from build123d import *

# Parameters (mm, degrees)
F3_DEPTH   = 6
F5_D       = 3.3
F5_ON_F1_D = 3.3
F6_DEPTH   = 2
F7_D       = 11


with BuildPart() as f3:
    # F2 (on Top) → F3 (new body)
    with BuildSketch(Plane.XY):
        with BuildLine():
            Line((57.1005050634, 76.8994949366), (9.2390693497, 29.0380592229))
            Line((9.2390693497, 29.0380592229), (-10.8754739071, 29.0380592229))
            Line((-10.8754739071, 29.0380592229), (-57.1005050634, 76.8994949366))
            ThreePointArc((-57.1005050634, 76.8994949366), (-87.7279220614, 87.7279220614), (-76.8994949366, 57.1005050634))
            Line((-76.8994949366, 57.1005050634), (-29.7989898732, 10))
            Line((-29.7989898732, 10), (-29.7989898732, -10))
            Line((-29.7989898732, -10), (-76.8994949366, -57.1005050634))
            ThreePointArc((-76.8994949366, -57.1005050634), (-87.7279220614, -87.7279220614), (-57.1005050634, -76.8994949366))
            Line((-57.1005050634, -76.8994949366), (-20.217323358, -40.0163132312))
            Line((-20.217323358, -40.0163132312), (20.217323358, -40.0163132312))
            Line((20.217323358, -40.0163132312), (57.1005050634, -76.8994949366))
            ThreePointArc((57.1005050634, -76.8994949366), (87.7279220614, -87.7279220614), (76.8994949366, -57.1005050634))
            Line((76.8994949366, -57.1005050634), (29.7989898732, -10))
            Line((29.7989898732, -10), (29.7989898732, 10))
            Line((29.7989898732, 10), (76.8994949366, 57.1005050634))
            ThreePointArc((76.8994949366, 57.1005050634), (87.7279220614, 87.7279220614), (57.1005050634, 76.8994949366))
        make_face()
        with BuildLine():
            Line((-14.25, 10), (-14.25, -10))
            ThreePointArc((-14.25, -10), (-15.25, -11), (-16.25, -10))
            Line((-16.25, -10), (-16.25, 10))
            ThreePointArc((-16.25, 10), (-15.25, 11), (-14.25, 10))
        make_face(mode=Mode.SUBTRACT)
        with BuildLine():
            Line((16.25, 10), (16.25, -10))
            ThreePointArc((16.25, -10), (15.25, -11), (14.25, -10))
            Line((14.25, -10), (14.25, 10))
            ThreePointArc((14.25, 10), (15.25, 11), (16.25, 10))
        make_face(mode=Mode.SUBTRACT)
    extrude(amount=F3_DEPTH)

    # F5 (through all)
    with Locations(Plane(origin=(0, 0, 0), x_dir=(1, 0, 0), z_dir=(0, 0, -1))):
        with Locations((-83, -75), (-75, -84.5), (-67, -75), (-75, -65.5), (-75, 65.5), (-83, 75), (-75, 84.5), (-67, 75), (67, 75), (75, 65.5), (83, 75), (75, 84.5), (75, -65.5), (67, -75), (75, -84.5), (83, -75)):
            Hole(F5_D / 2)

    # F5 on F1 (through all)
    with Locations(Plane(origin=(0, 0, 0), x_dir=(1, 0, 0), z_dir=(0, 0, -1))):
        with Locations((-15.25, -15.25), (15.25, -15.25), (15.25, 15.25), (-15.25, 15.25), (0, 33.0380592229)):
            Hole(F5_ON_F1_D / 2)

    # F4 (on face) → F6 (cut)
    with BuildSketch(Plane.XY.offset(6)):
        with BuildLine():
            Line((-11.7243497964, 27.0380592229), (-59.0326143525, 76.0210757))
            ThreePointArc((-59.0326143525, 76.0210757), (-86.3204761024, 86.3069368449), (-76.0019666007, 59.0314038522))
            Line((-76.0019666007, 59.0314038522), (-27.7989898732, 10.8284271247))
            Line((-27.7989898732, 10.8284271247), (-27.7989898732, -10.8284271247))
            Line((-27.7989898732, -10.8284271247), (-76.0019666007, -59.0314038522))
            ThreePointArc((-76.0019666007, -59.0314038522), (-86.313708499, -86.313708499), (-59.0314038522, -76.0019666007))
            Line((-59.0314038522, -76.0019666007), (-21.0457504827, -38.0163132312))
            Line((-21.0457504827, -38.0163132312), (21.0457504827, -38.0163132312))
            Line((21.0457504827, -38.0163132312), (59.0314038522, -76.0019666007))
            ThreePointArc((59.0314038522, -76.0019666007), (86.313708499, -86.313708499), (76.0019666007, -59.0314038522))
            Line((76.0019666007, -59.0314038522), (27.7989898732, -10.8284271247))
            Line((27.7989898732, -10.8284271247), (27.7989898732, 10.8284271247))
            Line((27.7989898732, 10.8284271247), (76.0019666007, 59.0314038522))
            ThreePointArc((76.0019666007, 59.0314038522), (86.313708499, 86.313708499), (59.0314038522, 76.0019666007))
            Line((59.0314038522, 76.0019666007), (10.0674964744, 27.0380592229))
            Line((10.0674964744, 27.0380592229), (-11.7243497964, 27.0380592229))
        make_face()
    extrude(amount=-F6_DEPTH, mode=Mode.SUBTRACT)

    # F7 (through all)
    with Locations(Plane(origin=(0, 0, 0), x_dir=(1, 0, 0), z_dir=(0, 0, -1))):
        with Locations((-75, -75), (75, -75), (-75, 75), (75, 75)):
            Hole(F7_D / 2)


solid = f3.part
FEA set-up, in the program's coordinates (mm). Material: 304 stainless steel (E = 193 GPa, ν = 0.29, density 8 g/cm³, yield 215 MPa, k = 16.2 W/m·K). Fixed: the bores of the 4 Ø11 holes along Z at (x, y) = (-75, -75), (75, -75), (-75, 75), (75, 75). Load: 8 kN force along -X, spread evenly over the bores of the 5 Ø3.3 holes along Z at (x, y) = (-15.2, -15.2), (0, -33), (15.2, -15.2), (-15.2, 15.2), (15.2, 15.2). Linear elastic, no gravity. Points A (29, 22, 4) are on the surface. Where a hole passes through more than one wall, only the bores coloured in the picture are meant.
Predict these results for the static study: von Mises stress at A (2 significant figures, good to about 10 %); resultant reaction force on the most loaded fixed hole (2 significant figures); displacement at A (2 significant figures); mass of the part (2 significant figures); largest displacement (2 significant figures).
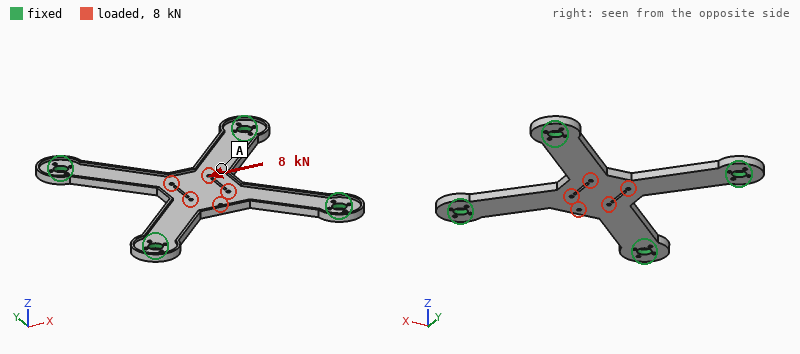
18 MPa
2.8 kN
11 µm
460 g
17 µm
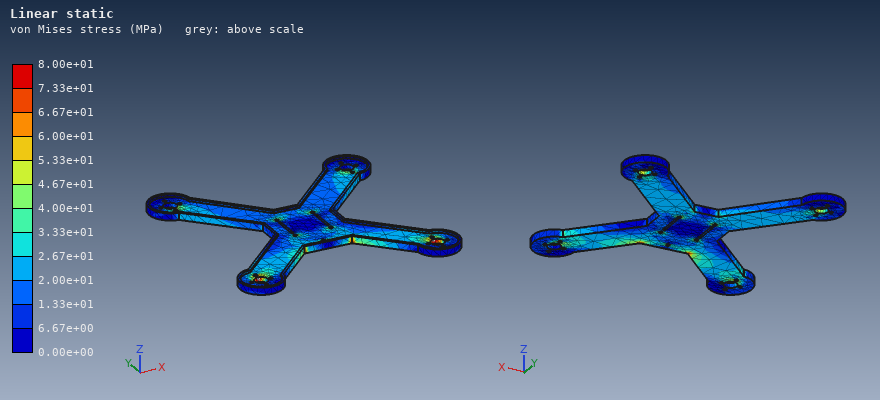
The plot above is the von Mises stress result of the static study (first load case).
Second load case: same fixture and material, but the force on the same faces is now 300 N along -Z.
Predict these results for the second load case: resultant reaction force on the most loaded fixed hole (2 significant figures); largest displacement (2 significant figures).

84 N
0.12 mm
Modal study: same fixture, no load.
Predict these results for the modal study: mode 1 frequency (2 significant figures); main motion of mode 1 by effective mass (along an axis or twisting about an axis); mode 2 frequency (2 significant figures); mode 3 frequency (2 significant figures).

620 Hz
along Z
1500 Hz
1500 Hz
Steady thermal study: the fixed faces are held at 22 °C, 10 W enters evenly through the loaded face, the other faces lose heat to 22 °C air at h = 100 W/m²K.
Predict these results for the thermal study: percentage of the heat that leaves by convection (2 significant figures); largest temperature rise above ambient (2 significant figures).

99 %
19 K
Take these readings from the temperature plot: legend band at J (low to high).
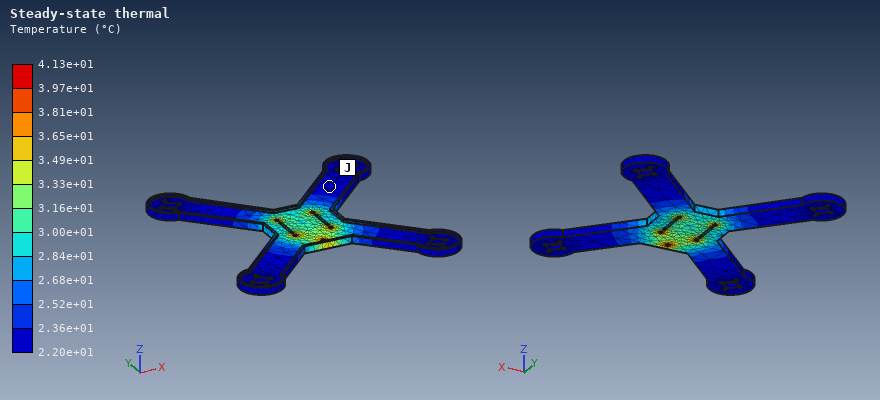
2.20e+01 to 2.36e+01 °C
